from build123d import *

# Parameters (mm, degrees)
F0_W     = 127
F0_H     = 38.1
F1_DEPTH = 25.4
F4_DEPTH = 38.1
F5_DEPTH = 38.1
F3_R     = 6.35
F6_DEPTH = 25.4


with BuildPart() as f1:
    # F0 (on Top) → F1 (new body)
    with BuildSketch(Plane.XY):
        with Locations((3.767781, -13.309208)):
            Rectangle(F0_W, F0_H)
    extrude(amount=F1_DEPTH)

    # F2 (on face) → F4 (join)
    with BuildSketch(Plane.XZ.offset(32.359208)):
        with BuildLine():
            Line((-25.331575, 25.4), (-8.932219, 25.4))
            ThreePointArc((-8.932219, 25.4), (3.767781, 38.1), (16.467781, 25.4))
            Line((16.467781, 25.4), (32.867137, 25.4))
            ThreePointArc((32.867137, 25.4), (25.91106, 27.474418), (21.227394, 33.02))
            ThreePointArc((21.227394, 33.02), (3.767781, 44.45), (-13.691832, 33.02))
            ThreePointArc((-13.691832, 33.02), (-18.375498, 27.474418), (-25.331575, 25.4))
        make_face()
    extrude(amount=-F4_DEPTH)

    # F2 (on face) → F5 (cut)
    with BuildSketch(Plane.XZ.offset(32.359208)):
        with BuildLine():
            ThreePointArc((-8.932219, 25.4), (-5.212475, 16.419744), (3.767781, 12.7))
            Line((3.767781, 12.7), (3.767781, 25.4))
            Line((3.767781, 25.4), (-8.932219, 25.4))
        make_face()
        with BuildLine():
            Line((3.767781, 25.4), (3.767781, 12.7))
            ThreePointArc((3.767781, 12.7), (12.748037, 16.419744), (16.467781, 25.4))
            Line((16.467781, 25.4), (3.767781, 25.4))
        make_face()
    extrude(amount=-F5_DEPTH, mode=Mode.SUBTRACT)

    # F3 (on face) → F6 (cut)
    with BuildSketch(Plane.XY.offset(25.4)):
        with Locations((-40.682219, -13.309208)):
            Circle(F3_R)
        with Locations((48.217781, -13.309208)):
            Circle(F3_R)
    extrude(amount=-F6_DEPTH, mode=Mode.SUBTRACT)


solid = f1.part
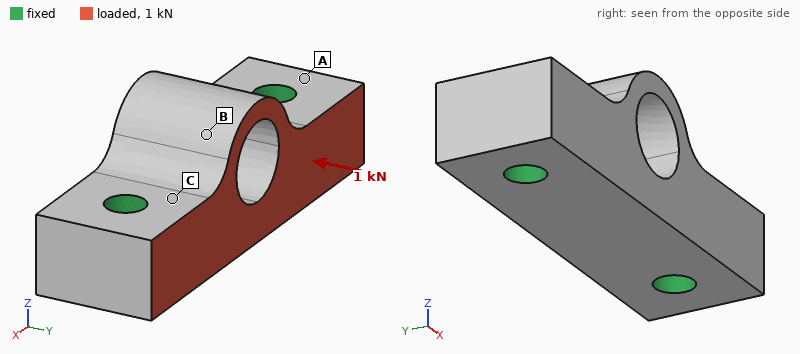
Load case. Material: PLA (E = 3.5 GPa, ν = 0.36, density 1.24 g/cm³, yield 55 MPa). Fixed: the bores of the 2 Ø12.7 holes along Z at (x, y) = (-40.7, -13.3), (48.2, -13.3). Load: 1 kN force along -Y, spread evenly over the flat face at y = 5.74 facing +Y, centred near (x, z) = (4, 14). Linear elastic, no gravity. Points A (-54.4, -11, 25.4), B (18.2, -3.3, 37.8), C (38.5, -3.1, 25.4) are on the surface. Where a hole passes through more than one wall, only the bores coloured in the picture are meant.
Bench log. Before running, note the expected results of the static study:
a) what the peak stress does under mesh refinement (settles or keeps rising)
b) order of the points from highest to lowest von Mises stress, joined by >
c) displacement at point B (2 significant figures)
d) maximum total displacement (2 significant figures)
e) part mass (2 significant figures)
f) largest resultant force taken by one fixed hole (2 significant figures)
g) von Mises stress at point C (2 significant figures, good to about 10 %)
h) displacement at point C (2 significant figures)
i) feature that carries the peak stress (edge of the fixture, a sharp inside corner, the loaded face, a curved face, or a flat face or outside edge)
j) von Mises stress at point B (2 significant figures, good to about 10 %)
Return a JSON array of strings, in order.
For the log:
["keeps rising", "C > B > A", "17 µm", "24 µm", "150 g", "500 N", "0.79 MPa", "4.5 µm", "edge of the fixture", "0.50 MPa"]
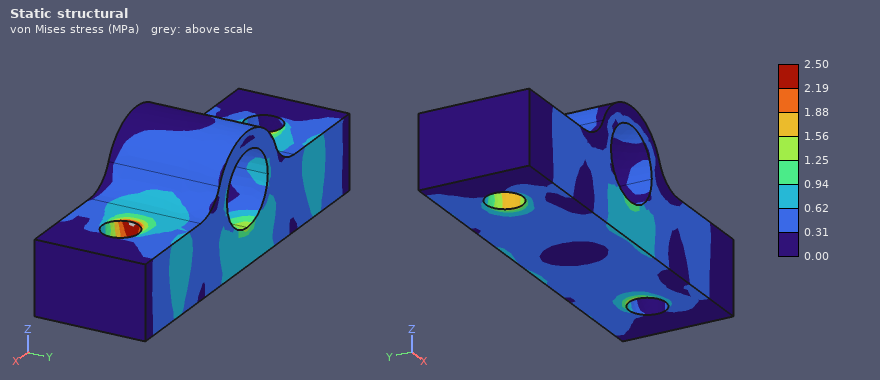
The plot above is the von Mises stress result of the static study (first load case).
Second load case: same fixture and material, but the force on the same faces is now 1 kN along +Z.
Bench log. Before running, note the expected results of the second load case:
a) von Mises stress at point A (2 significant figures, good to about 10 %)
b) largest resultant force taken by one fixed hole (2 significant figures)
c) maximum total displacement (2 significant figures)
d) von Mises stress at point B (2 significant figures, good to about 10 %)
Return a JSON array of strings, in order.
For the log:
["0.57 MPa", "500 N", "43 µm", "0.60 MPa"]
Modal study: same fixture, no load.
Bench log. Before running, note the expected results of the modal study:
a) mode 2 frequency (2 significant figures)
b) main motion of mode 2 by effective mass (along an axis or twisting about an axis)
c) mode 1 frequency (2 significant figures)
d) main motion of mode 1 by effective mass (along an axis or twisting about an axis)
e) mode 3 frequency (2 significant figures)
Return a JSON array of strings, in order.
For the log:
["4000 Hz", "along Z", "3400 Hz", "along Y", "4400 Hz"]
